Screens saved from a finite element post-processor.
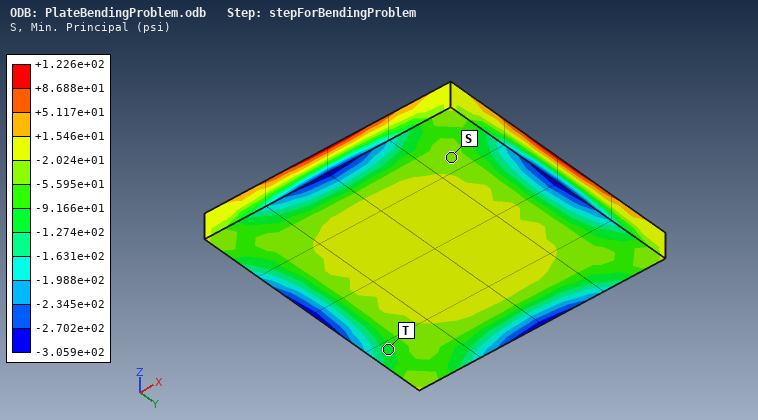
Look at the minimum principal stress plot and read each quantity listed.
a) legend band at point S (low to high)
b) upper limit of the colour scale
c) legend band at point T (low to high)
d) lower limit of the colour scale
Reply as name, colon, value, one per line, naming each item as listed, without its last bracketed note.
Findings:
legend band at point S: -5.595e+01 to -2.024e+01 psi
upper limit of the colour scale: +1.226e+02 psi
legend band at point T: -1.274e+02 to -9.166e+01 psi
lower limit of the colour scale: -3.059e+02 psi
